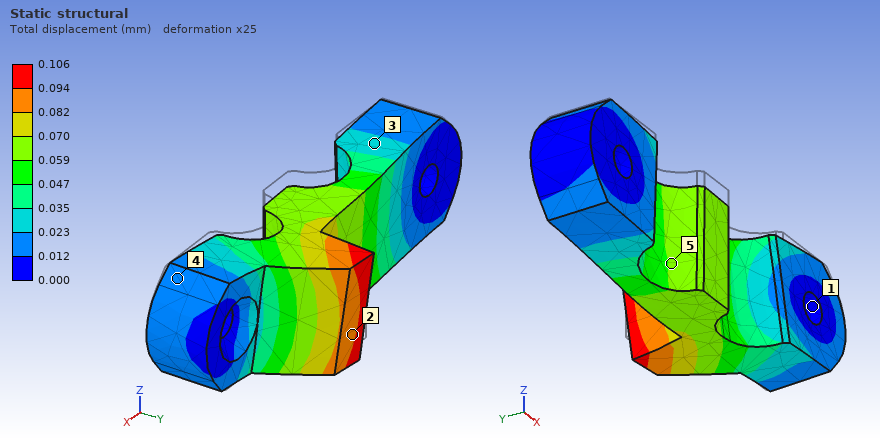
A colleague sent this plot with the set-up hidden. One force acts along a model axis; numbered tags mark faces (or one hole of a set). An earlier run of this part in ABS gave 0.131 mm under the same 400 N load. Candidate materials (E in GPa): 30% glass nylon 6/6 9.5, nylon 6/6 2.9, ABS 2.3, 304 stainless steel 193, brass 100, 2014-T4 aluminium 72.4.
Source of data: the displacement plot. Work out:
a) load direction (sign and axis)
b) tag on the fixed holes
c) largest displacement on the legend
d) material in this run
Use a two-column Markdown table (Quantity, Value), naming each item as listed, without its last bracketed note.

| Quantity | Value |
|---|---|
| load direction | -Z |
| tag on the fixed holes | 1 |
| largest displacement on the legend | 0.106 mm |
| material in this run | nylon 6/6 |
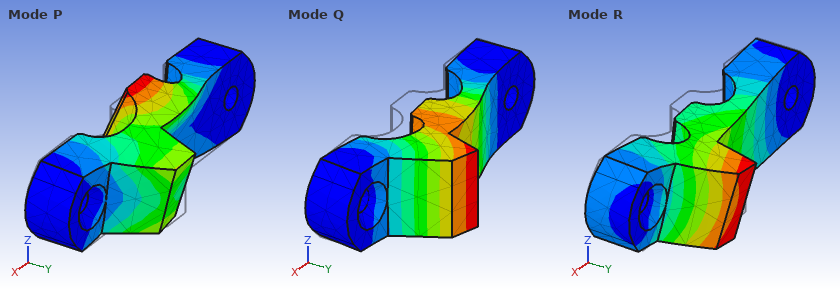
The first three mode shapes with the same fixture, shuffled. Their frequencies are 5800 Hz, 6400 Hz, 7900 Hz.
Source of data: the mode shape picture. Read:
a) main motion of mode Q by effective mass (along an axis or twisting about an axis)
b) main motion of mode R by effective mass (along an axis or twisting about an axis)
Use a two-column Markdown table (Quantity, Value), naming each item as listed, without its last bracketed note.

| Quantity | Value |
|---|---|
| main motion of mode Q by effective mass | along Y |
| main motion of mode R by effective mass | along Z |
